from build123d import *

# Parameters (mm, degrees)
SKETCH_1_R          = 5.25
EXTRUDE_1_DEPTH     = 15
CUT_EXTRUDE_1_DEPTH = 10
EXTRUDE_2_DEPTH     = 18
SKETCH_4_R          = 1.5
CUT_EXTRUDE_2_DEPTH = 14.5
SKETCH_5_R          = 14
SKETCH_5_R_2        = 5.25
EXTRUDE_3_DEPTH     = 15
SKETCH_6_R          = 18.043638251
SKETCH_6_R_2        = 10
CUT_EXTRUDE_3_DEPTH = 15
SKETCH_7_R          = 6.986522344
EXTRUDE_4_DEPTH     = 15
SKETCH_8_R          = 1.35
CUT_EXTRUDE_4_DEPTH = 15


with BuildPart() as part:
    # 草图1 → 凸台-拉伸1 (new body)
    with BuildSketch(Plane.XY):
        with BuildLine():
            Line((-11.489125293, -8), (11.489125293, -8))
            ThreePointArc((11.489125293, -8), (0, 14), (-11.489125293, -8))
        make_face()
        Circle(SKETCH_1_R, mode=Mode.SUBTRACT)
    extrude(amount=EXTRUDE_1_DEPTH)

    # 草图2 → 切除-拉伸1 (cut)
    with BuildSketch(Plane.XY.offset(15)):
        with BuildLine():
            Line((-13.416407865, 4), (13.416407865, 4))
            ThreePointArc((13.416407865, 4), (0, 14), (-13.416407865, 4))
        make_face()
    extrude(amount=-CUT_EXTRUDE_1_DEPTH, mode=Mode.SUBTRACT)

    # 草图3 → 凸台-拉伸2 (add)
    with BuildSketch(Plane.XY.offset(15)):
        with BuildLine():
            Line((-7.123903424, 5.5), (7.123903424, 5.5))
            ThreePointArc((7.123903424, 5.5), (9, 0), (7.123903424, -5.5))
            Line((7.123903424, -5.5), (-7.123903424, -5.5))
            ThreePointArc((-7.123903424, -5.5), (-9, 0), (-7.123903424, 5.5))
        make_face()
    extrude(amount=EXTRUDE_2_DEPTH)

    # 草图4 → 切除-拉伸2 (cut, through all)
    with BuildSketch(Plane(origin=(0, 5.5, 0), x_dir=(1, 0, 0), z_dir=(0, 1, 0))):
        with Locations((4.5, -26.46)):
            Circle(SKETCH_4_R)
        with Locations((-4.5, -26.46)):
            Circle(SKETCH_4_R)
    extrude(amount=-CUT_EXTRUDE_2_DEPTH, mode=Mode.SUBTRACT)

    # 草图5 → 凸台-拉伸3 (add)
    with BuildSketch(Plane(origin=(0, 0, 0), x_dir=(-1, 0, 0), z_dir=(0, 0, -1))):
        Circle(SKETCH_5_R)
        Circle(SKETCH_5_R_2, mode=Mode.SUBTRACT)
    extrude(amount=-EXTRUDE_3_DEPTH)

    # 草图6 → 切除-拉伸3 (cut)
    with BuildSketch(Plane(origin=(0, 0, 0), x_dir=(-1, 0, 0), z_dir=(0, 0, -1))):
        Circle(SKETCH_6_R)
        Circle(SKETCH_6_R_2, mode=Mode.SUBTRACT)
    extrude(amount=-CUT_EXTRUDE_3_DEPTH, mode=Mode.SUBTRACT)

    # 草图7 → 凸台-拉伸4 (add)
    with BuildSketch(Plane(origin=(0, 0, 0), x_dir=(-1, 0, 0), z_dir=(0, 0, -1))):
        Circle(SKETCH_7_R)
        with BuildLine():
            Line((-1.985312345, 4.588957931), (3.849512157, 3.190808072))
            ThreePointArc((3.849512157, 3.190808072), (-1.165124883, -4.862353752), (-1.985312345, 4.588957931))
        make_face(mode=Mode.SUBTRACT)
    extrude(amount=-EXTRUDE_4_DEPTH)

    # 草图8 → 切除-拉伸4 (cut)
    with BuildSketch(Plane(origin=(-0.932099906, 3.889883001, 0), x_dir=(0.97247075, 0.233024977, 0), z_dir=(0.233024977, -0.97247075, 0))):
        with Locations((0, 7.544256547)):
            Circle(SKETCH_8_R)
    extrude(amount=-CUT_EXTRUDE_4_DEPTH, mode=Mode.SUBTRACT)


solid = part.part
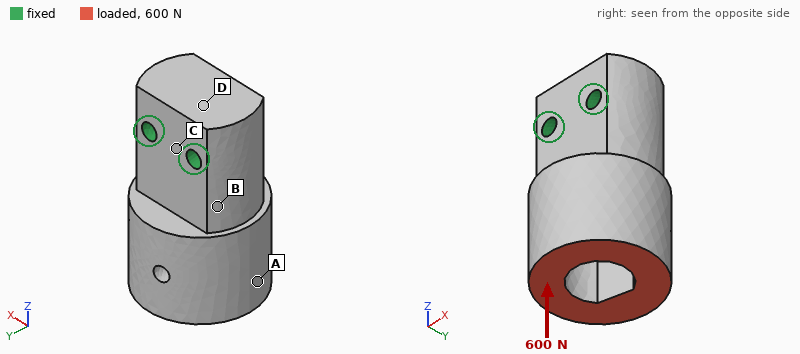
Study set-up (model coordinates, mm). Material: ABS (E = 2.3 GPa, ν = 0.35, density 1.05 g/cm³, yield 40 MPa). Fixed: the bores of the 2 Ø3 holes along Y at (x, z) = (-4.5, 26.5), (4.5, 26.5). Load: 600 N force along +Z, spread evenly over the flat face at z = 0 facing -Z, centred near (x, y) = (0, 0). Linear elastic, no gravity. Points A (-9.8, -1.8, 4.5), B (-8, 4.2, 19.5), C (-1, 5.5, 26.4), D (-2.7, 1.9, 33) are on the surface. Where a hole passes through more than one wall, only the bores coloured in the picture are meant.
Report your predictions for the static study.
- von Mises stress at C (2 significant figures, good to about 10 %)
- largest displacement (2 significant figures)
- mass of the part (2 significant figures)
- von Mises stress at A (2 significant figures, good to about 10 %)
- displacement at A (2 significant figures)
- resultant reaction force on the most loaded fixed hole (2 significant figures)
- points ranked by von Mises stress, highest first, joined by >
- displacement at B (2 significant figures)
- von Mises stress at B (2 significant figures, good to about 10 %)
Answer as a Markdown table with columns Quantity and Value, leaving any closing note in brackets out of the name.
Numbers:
| Quantity | Value |
|---|---|
| von Mises stress at C | 1.3 MPa |
| largest displacement | 44 µm |
| mass of the part | 7.1 g |
| von Mises stress at A | 2.6 MPa |
| displacement at A | 32 µm |
| resultant reaction force on the most loaded fixed hole | 300 N |
| points ranked by von Mises stress, highest first, joined by > | B > A > C > D |
| displacement at B | 12 µm |
| von Mises stress at B | 3.8 MPa |
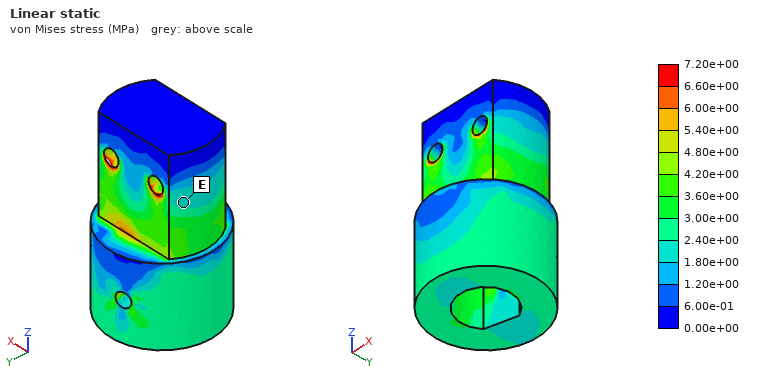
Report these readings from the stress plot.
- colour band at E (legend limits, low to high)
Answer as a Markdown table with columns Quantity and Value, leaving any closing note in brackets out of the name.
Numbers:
| Quantity | Value |
|---|---|
| colour band at E | 1.80e+00 to 2.40e+00 MPa |
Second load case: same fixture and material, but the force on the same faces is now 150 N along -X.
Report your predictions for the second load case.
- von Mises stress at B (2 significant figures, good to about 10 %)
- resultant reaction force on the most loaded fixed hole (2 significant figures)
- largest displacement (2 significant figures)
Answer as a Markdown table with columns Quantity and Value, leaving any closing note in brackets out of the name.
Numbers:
| Quantity | Value |
|---|---|
| von Mises stress at B | 5.5 MPa |
| resultant reaction force on the most loaded fixed hole | 370 N |
| largest displacement | 0.15 mm |
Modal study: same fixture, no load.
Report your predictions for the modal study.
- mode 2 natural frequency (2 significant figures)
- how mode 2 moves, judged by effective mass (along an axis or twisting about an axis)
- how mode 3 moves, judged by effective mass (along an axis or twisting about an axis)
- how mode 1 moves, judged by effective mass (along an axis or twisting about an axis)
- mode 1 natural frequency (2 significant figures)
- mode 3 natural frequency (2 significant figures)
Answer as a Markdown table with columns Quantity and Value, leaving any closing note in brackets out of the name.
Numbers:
| Quantity | Value |
|---|---|
| mode 2 natural frequency | 3800 Hz |
| how mode 2 moves, judged by effective mass | along X |
| how mode 3 moves, judged by effective mass | twisting about Z |
| how mode 1 moves, judged by effective mass | along Y |
| mode 1 natural frequency | 2800 Hz |
| mode 3 natural frequency | 5800 Hz |
